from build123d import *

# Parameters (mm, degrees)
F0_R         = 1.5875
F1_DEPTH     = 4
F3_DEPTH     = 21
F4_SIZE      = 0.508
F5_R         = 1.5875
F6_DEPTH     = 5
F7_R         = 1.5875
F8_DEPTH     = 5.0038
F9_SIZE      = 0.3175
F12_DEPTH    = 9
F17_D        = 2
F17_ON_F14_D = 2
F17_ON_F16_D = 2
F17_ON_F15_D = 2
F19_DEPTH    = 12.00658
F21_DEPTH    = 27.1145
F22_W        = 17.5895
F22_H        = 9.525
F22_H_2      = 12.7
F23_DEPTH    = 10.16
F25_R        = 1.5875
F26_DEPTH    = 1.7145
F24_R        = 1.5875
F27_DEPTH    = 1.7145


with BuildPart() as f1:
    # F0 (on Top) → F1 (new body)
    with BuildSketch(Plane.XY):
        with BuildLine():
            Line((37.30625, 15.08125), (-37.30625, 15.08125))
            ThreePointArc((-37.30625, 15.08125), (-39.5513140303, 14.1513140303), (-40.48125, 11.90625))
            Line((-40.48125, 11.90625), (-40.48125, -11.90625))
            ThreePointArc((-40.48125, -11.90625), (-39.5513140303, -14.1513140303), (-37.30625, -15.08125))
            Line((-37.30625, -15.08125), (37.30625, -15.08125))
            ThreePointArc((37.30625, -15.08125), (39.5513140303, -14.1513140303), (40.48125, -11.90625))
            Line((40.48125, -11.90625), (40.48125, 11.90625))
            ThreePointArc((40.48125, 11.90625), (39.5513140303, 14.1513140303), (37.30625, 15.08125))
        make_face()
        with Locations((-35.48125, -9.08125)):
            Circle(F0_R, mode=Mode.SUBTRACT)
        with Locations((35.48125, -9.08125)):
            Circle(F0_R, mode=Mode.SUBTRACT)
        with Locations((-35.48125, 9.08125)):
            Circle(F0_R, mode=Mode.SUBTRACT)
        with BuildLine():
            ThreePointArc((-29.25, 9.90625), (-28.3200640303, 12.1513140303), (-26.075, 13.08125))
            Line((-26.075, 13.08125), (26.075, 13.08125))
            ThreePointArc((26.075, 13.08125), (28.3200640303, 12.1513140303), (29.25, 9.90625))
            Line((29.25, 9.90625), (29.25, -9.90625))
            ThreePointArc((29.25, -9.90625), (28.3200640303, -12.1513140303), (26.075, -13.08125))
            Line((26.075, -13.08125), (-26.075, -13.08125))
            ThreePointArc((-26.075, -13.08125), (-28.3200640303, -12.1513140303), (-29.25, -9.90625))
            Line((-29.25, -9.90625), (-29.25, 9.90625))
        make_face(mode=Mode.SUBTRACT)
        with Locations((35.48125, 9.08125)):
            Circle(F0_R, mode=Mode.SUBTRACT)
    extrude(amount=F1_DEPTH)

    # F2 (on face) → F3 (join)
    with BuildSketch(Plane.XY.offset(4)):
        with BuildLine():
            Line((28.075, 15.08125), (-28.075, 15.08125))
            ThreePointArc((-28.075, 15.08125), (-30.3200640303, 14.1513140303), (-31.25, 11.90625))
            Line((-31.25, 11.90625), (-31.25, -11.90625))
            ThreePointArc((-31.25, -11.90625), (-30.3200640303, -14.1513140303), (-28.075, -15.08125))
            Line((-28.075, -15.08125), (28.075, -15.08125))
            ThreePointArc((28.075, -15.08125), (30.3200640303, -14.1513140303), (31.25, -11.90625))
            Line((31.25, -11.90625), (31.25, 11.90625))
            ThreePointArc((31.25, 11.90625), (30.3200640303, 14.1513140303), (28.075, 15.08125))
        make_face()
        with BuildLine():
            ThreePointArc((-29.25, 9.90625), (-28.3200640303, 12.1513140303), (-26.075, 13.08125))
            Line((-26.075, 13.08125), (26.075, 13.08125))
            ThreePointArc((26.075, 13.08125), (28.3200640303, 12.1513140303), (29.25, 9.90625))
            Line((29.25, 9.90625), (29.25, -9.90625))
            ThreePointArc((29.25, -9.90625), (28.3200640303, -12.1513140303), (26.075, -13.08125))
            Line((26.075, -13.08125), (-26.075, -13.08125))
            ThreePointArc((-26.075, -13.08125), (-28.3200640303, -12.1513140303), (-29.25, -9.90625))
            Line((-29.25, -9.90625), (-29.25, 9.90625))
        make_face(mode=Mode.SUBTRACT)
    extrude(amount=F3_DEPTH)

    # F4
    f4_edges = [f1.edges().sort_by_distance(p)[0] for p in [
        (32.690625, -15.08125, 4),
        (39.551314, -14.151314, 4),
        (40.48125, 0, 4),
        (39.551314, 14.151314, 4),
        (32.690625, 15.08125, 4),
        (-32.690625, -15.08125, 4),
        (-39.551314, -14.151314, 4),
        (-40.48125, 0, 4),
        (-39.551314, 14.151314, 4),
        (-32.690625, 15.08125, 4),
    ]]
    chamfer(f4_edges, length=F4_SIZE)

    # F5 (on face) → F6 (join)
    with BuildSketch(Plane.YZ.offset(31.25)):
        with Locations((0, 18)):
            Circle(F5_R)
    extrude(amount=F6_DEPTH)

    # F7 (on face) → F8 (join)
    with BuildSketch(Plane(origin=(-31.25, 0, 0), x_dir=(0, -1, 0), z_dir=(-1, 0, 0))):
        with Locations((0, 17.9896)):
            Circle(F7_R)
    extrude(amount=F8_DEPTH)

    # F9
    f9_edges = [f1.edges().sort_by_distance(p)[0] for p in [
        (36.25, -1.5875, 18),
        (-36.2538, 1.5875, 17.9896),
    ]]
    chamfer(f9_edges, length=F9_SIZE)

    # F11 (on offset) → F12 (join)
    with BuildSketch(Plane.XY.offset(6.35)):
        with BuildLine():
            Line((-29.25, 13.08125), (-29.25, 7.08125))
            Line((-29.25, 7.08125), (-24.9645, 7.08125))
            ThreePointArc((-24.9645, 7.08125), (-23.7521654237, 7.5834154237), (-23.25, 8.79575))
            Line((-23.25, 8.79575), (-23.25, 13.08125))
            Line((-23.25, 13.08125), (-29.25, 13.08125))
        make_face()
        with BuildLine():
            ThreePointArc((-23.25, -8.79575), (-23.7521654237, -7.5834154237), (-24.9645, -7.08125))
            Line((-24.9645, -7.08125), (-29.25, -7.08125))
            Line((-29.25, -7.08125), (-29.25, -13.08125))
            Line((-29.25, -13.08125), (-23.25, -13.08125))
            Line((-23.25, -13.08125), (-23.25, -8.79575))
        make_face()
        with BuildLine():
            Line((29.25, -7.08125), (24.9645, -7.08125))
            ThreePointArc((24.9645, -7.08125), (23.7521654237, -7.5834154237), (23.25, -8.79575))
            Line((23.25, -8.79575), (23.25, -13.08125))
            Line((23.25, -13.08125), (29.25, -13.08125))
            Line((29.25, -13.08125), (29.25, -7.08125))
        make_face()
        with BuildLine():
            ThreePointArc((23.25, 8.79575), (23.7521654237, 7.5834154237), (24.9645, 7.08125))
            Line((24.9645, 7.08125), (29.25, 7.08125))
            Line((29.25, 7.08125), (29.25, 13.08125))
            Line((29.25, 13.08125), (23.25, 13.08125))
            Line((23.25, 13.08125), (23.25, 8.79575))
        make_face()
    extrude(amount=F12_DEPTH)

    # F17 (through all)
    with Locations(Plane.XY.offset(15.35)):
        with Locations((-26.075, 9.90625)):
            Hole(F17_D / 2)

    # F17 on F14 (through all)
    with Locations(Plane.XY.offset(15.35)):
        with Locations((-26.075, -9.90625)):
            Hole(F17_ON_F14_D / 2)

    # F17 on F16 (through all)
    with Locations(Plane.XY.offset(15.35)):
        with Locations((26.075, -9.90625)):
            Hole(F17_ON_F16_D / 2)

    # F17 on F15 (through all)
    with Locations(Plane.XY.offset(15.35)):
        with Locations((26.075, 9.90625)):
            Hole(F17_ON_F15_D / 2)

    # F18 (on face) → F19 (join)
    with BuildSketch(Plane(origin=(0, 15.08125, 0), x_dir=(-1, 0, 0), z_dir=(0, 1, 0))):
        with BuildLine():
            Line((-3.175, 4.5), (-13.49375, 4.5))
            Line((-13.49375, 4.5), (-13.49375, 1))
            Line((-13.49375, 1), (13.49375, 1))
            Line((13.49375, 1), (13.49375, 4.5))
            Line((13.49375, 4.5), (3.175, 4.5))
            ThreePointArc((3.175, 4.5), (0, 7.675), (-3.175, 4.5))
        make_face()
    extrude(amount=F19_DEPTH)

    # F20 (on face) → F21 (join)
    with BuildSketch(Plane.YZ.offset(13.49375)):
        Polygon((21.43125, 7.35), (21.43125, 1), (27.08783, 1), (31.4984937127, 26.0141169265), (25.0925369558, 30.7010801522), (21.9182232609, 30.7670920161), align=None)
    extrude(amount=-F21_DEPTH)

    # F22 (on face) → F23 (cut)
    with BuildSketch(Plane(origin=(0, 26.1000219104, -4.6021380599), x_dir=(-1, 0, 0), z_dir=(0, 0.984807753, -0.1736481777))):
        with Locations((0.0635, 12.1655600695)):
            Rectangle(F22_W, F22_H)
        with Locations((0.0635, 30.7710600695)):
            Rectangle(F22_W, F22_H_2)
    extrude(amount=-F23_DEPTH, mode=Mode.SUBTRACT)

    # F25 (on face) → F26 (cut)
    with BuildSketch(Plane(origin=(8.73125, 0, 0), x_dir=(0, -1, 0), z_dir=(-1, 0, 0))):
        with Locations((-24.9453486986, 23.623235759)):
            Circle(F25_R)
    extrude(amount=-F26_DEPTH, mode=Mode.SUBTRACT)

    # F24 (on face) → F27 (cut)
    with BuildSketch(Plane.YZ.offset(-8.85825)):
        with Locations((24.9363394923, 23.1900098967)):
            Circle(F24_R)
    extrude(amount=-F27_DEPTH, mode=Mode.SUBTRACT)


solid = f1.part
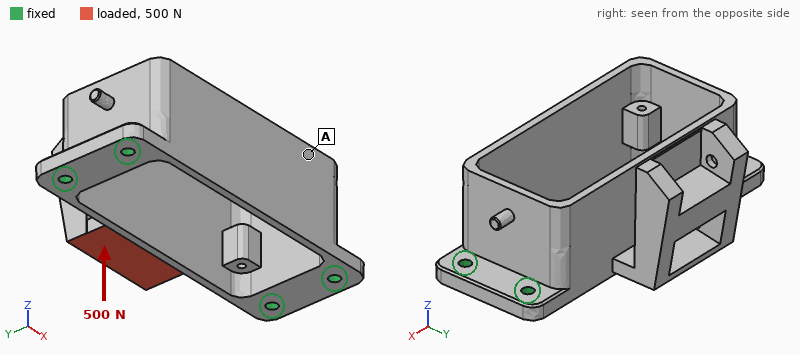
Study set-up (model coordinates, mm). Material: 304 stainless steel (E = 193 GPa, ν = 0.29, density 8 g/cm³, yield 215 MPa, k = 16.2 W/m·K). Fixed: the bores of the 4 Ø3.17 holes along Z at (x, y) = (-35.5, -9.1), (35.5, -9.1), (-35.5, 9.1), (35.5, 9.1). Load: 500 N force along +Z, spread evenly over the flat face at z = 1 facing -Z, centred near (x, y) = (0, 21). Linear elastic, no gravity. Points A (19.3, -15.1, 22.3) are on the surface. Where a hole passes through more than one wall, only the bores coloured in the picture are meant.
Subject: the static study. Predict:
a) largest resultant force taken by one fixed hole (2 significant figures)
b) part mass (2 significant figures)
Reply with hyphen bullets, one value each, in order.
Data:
- 460 N
- 130 g
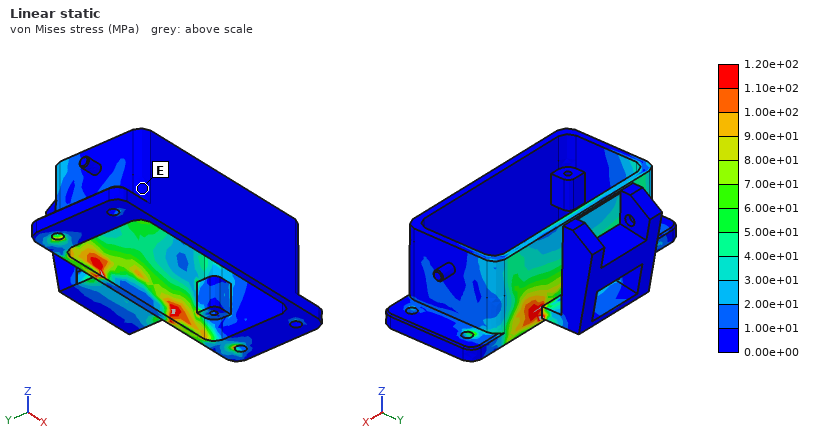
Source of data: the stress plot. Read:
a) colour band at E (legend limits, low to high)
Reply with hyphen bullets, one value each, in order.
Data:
- 0.00e+00 to 1.00e+01 MPa
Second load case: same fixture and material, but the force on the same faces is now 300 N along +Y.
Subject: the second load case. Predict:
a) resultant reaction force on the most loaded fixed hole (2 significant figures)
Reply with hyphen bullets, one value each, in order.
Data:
- 180 N
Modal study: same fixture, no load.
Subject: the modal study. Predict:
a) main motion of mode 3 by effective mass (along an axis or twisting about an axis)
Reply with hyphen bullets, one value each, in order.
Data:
- along Y
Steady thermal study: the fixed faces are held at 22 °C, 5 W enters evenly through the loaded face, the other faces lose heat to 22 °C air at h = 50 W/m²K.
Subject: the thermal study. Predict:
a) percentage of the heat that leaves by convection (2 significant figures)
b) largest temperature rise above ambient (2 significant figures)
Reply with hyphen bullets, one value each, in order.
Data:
- 89 %
- 41 K
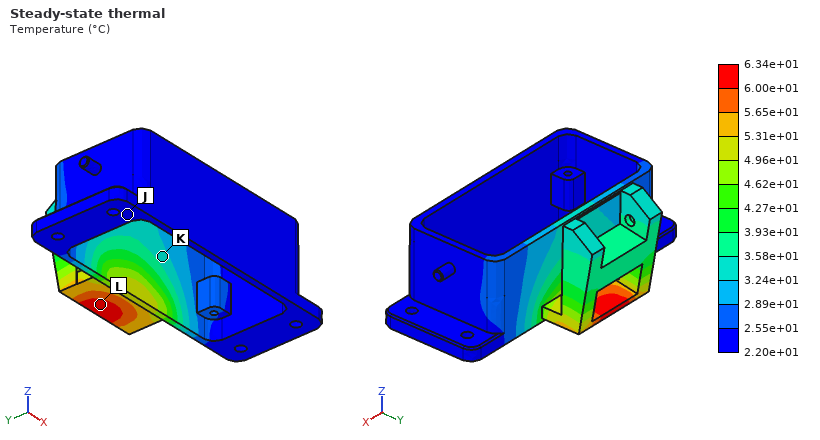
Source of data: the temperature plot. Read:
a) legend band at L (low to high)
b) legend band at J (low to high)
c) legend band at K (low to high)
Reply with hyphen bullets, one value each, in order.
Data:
- 6.00e+01 to 6.34e+01 °C
- 2.20e+01 to 2.55e+01 °C
- 3.24e+01 to 3.58e+01 °C
